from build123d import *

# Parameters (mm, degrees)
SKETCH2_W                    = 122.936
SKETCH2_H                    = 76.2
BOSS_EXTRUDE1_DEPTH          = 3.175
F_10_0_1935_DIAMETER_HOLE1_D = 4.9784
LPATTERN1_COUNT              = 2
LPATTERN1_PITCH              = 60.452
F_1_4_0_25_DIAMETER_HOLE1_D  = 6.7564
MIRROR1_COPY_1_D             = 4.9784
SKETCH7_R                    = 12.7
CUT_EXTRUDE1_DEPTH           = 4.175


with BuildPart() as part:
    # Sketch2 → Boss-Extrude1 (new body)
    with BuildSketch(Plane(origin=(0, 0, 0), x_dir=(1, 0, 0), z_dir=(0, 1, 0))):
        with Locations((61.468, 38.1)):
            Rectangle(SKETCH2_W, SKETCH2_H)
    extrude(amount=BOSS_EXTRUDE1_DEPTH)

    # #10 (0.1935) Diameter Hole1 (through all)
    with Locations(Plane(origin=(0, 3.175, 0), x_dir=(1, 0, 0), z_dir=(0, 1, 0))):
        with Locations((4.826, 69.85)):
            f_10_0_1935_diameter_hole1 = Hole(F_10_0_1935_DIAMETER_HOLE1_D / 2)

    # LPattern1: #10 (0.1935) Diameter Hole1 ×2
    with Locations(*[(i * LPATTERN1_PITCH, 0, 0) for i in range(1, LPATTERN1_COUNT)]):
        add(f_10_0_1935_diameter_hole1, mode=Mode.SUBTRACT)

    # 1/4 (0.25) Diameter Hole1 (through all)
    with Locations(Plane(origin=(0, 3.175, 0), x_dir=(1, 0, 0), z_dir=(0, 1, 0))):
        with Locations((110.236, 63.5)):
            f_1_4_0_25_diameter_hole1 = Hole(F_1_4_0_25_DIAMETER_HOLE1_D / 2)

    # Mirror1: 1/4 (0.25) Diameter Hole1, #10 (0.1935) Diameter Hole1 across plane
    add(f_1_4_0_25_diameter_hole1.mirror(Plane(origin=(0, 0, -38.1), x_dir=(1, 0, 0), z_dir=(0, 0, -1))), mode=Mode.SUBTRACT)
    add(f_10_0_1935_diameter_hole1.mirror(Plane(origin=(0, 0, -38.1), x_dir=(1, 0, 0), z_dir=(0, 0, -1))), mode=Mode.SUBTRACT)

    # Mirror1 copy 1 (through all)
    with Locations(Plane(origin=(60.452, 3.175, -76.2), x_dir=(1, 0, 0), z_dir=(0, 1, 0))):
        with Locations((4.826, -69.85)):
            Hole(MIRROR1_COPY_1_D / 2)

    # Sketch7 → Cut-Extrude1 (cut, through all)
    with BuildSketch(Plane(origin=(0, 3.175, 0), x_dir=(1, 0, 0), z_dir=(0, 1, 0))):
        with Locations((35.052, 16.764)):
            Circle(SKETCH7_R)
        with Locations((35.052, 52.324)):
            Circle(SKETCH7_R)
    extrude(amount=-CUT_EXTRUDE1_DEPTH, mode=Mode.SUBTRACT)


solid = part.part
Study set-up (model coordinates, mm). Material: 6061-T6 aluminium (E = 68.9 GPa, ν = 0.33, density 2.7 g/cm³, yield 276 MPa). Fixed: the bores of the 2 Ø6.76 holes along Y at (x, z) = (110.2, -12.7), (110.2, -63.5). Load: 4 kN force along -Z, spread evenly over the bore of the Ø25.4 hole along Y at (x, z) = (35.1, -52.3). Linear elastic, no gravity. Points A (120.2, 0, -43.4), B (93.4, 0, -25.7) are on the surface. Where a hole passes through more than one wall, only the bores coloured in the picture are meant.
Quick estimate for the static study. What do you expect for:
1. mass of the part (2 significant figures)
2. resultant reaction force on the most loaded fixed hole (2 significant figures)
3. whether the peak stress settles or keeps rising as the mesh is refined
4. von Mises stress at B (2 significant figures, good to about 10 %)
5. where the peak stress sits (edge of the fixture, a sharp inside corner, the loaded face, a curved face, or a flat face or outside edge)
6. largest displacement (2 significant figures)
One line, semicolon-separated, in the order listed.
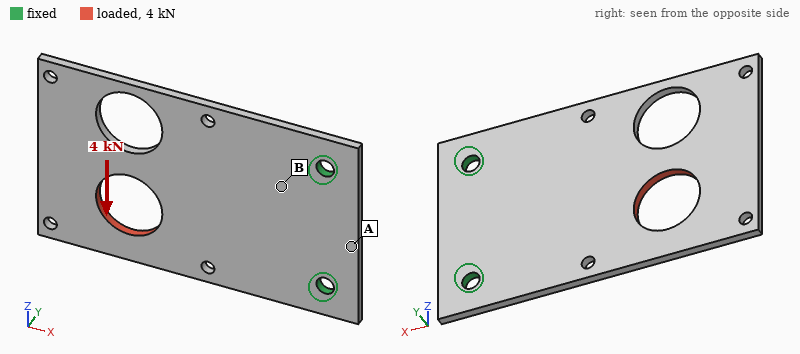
70 g; 5.9 kN; keeps rising; 52 MPa; edge of the fixture; 0.27 mm
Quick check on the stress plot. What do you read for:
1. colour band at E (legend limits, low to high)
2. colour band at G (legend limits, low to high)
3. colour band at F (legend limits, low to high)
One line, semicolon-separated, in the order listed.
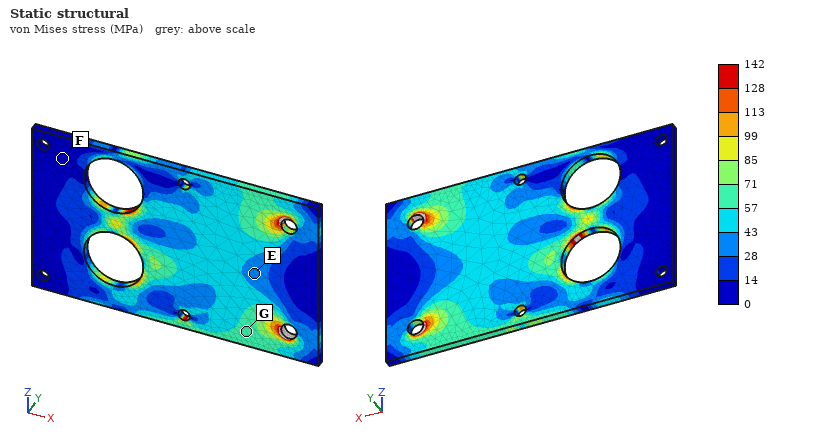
28 to 43 MPa; 57 to 71 MPa; 0 to 14 MPa
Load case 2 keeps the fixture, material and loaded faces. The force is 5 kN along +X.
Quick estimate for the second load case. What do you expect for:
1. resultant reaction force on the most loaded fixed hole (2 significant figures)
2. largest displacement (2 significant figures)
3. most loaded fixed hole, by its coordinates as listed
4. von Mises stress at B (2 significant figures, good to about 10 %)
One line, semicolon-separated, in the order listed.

3.9 kN; 80 µm; (110.2, -63.5); 12 MPa
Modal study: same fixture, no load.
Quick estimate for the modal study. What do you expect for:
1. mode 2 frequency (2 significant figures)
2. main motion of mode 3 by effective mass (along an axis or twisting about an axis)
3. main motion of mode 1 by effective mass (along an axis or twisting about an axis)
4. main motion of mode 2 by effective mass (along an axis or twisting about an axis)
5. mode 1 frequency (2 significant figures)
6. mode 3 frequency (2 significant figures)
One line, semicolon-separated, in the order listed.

710 Hz; along Y; along Y; twisting about X; 230 Hz; 1200 Hz
